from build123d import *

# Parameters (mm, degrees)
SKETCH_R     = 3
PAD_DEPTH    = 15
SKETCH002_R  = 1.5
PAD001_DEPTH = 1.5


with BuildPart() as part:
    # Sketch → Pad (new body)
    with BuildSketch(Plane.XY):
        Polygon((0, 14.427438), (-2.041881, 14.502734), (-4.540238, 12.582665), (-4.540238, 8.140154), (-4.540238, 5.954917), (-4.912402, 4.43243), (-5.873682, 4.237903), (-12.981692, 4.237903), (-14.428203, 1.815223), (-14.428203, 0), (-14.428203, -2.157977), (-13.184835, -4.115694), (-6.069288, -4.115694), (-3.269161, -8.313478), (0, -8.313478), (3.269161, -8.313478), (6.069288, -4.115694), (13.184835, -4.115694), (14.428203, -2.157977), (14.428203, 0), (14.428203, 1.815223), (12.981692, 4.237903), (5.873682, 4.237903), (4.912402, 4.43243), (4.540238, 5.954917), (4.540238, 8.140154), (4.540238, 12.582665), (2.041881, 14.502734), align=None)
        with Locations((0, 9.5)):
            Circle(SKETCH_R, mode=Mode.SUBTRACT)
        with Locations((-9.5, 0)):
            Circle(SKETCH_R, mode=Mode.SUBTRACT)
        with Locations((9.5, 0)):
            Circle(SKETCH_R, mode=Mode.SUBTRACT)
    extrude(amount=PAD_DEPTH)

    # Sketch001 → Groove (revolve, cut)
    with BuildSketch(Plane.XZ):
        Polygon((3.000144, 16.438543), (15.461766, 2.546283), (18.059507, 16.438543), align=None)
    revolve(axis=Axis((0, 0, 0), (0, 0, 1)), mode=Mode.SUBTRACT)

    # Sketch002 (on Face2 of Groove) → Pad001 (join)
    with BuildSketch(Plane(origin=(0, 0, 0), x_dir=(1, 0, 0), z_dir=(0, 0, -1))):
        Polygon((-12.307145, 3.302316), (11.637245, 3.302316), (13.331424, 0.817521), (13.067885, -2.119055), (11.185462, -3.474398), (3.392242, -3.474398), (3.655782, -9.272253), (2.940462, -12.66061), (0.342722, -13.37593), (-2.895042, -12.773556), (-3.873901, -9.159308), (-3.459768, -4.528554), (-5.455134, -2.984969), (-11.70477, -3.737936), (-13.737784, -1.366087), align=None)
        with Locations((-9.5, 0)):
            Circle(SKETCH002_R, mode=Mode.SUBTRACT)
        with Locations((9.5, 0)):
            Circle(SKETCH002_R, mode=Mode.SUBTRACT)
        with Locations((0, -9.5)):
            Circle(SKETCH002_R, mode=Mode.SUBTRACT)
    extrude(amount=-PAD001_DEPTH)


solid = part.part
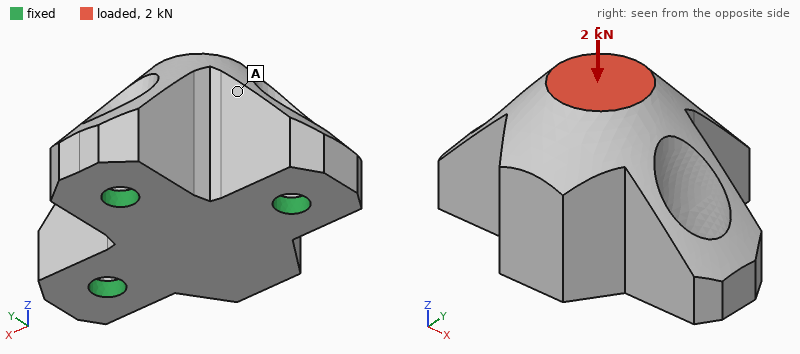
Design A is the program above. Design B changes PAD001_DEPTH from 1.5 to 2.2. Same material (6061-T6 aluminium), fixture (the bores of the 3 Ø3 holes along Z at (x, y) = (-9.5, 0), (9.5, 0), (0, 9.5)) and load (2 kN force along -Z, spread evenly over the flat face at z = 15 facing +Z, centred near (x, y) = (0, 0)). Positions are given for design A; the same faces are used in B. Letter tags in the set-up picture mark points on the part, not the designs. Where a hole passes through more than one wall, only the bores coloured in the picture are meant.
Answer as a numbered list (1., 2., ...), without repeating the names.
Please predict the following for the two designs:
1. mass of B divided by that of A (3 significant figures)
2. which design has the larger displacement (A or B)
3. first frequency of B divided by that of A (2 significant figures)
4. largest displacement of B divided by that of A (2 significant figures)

1. 1.01
2. A
3. 1.2
4. 0.70
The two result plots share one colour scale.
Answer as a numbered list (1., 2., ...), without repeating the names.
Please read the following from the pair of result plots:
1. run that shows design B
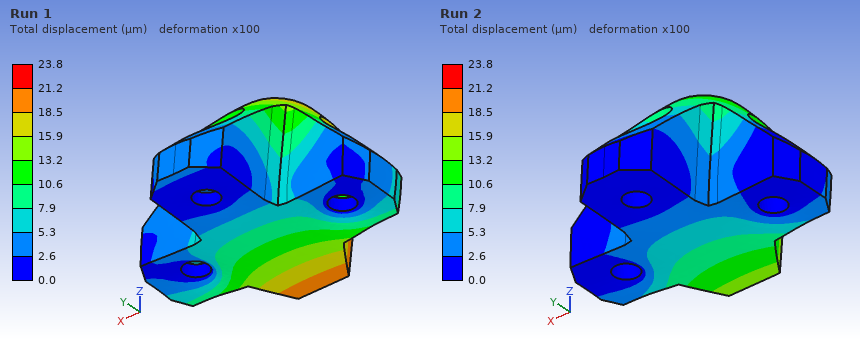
1. Run 2
